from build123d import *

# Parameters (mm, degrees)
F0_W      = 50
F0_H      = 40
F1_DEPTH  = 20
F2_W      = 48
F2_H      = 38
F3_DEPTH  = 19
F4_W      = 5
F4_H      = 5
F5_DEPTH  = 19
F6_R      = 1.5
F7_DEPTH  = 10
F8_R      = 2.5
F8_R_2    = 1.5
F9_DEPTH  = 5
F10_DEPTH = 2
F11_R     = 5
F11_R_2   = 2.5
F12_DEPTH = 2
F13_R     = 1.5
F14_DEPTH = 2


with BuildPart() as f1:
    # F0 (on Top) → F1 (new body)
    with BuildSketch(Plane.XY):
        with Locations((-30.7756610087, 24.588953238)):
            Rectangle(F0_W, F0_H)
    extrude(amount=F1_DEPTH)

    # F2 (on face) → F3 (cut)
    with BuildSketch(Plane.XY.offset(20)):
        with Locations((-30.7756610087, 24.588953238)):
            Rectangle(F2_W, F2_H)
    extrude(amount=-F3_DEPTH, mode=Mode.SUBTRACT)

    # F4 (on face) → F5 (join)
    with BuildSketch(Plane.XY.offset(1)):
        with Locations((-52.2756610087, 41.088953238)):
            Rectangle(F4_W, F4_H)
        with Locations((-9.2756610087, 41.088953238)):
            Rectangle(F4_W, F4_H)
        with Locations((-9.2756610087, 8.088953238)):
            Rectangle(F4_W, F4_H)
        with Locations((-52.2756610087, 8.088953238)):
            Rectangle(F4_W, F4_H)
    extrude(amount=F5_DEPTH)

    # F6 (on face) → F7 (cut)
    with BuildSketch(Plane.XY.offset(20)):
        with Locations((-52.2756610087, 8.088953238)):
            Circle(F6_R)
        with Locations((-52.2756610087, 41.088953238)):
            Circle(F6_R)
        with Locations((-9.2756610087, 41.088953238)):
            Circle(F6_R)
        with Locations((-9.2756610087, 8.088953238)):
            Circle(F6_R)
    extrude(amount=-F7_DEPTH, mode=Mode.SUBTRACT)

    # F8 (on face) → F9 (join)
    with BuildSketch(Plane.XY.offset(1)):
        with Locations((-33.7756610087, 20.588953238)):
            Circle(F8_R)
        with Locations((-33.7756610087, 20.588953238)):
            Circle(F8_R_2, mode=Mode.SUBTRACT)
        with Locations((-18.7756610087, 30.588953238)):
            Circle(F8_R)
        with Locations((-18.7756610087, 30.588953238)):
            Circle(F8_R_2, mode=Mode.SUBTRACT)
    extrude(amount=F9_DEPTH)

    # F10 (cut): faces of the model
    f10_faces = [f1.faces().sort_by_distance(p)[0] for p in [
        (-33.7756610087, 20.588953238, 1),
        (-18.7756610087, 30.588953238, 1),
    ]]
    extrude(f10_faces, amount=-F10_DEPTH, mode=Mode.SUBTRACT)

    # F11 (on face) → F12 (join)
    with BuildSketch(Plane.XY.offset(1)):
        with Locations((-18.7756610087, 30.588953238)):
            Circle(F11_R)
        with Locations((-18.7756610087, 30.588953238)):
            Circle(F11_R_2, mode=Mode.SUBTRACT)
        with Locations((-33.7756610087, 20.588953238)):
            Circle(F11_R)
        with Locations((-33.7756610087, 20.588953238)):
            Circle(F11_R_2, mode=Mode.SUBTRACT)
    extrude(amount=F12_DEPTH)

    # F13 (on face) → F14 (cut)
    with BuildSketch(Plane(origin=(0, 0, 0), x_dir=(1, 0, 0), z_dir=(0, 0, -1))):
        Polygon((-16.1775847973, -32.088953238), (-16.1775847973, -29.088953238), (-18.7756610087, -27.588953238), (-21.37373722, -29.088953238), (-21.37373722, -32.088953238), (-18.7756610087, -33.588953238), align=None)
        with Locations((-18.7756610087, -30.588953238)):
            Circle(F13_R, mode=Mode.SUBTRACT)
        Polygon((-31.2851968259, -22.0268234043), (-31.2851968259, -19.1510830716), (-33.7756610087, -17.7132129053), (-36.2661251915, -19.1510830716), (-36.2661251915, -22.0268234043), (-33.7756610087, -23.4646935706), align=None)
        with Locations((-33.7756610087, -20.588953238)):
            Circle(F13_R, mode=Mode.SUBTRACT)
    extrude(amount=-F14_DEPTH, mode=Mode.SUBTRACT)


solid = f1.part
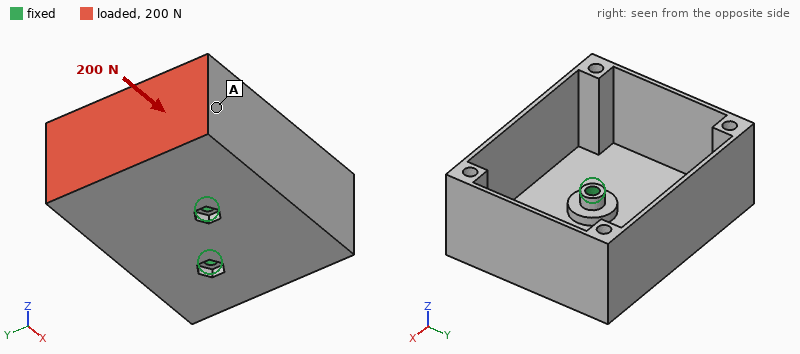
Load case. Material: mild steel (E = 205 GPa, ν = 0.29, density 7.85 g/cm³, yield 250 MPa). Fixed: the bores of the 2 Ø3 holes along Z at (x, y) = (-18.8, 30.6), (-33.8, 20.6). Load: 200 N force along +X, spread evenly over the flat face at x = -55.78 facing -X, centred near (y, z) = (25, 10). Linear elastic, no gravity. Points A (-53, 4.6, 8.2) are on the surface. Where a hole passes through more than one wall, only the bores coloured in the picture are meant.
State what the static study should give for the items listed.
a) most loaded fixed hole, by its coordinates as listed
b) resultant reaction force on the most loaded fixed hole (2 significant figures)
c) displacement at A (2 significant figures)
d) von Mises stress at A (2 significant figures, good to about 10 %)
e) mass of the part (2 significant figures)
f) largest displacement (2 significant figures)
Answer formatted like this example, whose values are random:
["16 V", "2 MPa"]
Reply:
["(-33.8, 20.6)", "120 N", "0.043 mm", "13 MPa", "57 g", "0.10 mm"]
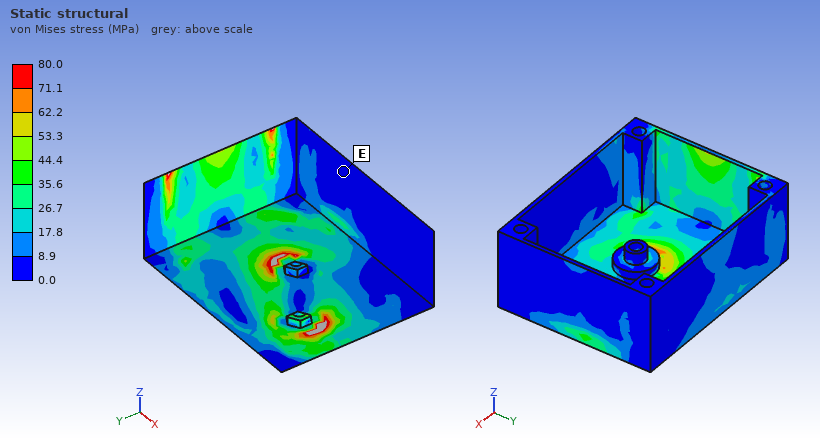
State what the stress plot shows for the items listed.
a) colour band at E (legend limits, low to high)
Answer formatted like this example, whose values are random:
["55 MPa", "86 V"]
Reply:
["0.0 to 8.9 MPa"]
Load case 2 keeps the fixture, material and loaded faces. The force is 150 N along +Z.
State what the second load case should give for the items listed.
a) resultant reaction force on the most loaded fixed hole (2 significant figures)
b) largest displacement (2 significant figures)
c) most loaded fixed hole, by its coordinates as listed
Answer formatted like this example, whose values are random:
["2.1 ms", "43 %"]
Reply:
["220 N", "0.27 mm", "(-33.8, 20.6)"]
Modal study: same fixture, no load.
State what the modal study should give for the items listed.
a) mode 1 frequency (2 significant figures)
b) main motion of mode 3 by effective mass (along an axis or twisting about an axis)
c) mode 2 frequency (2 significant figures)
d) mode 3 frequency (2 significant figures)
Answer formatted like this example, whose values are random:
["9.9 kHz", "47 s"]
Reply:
["810 Hz", "along Z", "1100 Hz", "1300 Hz"]
